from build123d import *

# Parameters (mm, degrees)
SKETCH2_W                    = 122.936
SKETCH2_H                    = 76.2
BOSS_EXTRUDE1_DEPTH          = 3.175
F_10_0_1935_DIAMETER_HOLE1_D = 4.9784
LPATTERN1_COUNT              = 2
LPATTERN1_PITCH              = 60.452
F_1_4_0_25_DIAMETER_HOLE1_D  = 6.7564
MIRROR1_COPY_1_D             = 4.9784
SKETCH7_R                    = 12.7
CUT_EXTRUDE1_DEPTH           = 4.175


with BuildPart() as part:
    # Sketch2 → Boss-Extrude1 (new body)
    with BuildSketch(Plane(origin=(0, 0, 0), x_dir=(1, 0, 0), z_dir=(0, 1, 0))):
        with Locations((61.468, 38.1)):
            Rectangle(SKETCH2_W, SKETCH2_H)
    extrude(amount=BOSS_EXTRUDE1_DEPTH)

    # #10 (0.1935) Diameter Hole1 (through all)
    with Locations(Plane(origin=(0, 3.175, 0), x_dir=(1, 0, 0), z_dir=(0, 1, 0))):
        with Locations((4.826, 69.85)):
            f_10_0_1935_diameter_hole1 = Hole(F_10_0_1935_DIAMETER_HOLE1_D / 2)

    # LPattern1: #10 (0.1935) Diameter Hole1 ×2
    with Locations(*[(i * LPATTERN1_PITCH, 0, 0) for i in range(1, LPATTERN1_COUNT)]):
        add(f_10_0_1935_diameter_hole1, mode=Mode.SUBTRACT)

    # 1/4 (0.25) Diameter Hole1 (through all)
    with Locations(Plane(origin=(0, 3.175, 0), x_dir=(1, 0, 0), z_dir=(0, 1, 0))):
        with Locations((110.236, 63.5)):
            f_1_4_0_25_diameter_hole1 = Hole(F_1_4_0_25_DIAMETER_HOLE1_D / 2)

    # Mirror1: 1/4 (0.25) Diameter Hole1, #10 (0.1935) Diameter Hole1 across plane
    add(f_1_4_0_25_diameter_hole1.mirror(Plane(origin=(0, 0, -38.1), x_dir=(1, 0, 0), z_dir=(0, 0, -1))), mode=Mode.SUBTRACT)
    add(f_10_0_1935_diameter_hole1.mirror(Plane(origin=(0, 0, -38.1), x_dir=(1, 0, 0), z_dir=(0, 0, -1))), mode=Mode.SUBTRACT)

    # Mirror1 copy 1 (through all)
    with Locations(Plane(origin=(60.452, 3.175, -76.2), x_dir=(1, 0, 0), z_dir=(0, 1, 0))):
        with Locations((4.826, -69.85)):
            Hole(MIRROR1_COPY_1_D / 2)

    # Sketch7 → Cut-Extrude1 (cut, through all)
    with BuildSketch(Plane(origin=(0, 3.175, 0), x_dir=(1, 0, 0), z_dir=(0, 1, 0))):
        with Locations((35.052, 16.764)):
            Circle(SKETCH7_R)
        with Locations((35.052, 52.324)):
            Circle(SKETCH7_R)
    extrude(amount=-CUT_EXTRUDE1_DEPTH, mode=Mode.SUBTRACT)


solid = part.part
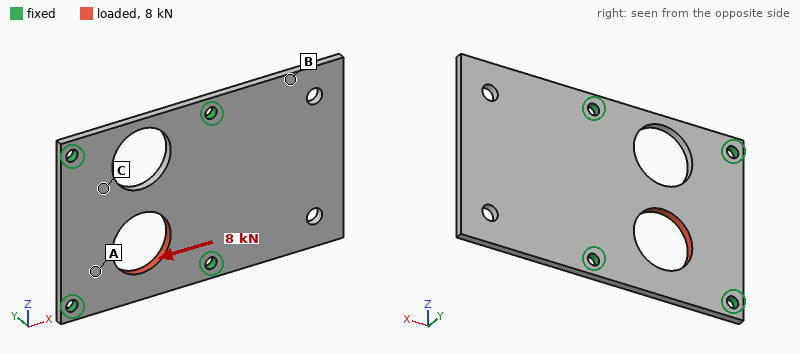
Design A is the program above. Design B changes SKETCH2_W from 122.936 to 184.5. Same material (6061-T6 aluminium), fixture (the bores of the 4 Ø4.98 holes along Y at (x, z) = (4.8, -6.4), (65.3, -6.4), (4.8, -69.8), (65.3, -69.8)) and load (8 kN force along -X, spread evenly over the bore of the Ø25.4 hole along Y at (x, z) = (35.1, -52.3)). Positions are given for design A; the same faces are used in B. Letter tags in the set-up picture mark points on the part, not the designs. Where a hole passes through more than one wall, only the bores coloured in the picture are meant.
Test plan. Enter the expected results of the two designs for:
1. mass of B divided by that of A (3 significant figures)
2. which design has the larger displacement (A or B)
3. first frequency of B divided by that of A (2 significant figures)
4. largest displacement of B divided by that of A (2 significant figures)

1.57
A
0.44
0.67
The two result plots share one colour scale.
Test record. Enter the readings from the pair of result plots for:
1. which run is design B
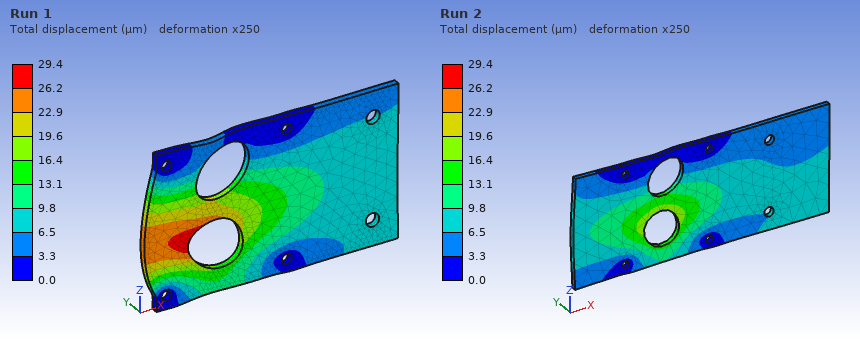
Run 2
